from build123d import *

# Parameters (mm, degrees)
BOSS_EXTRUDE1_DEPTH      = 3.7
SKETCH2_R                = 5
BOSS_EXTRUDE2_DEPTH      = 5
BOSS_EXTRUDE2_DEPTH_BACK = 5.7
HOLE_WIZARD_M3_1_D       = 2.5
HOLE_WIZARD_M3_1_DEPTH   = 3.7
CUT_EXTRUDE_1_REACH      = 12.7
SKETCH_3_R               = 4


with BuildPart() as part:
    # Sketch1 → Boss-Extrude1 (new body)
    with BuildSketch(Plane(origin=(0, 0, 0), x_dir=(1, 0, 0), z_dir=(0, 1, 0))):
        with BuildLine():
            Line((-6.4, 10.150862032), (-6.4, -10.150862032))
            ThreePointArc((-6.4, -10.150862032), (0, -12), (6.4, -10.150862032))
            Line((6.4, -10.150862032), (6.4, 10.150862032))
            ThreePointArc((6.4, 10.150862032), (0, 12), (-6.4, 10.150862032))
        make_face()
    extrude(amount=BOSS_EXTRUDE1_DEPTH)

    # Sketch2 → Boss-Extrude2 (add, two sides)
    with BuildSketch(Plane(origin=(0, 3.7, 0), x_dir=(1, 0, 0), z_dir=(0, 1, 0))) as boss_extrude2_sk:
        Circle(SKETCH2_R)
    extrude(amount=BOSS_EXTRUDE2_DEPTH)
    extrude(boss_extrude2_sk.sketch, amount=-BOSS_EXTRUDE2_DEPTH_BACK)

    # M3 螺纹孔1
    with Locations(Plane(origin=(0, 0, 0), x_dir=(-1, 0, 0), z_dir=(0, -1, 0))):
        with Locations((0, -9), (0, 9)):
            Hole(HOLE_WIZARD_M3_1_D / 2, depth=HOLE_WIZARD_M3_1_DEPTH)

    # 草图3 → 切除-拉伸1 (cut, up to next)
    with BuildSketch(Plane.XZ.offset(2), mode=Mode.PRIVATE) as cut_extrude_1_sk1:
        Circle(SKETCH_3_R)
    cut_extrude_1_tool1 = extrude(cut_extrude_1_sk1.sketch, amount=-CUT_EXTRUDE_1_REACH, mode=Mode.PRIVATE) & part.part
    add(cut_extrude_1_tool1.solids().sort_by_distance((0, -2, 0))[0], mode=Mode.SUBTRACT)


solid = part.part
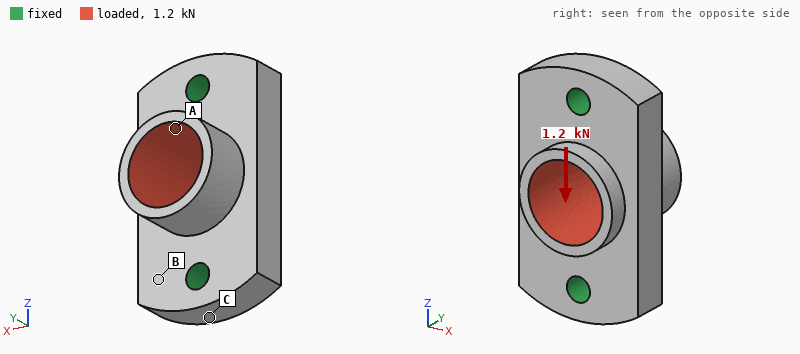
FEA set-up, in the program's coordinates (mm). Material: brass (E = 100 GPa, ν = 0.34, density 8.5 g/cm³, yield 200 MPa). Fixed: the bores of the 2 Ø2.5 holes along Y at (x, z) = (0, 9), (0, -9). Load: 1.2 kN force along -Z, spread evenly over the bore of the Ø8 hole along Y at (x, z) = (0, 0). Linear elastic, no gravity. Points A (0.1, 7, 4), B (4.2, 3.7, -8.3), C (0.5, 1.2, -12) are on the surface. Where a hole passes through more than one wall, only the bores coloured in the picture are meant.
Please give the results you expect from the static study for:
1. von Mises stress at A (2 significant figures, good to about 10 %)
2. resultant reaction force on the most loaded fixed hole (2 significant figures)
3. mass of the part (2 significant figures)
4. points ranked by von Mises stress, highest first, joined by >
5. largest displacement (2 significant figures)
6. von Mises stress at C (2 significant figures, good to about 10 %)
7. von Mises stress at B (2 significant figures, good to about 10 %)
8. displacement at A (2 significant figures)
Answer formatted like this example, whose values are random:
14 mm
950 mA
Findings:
27 MPa
610 N
9.0 g
A > C > B
6.6 µm
19 MPa
7.3 MPa
5.2 µm
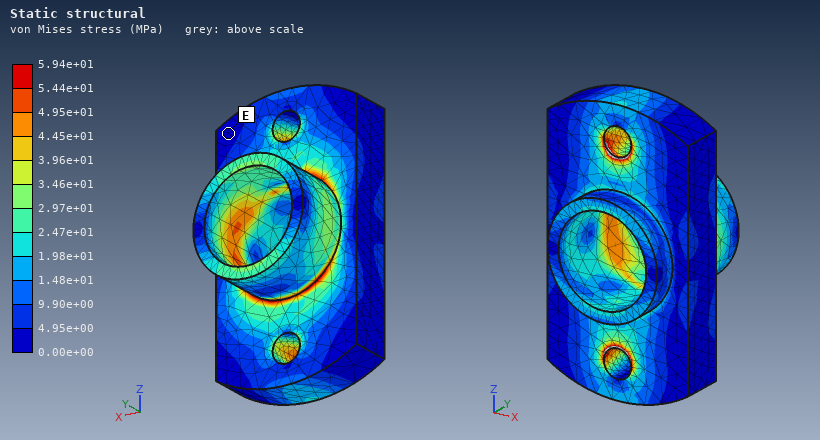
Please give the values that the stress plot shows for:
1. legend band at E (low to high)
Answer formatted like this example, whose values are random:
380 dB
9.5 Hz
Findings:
0.00e+00 to 4.95e+00 MPa
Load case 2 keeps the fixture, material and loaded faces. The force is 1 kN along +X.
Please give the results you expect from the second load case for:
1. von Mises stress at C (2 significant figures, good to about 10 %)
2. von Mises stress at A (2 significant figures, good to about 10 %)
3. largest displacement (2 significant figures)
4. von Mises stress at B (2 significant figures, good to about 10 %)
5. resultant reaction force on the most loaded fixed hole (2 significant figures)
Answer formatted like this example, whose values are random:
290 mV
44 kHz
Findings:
11 MPa
29 MPa
12 µm
17 MPa
500 N
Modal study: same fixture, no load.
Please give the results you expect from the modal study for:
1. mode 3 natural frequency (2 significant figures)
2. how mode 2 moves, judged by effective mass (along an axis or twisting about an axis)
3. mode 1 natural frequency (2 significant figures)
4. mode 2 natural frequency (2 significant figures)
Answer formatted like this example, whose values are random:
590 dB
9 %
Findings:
37 kHz
along Y
22 kHz
27 kHz
